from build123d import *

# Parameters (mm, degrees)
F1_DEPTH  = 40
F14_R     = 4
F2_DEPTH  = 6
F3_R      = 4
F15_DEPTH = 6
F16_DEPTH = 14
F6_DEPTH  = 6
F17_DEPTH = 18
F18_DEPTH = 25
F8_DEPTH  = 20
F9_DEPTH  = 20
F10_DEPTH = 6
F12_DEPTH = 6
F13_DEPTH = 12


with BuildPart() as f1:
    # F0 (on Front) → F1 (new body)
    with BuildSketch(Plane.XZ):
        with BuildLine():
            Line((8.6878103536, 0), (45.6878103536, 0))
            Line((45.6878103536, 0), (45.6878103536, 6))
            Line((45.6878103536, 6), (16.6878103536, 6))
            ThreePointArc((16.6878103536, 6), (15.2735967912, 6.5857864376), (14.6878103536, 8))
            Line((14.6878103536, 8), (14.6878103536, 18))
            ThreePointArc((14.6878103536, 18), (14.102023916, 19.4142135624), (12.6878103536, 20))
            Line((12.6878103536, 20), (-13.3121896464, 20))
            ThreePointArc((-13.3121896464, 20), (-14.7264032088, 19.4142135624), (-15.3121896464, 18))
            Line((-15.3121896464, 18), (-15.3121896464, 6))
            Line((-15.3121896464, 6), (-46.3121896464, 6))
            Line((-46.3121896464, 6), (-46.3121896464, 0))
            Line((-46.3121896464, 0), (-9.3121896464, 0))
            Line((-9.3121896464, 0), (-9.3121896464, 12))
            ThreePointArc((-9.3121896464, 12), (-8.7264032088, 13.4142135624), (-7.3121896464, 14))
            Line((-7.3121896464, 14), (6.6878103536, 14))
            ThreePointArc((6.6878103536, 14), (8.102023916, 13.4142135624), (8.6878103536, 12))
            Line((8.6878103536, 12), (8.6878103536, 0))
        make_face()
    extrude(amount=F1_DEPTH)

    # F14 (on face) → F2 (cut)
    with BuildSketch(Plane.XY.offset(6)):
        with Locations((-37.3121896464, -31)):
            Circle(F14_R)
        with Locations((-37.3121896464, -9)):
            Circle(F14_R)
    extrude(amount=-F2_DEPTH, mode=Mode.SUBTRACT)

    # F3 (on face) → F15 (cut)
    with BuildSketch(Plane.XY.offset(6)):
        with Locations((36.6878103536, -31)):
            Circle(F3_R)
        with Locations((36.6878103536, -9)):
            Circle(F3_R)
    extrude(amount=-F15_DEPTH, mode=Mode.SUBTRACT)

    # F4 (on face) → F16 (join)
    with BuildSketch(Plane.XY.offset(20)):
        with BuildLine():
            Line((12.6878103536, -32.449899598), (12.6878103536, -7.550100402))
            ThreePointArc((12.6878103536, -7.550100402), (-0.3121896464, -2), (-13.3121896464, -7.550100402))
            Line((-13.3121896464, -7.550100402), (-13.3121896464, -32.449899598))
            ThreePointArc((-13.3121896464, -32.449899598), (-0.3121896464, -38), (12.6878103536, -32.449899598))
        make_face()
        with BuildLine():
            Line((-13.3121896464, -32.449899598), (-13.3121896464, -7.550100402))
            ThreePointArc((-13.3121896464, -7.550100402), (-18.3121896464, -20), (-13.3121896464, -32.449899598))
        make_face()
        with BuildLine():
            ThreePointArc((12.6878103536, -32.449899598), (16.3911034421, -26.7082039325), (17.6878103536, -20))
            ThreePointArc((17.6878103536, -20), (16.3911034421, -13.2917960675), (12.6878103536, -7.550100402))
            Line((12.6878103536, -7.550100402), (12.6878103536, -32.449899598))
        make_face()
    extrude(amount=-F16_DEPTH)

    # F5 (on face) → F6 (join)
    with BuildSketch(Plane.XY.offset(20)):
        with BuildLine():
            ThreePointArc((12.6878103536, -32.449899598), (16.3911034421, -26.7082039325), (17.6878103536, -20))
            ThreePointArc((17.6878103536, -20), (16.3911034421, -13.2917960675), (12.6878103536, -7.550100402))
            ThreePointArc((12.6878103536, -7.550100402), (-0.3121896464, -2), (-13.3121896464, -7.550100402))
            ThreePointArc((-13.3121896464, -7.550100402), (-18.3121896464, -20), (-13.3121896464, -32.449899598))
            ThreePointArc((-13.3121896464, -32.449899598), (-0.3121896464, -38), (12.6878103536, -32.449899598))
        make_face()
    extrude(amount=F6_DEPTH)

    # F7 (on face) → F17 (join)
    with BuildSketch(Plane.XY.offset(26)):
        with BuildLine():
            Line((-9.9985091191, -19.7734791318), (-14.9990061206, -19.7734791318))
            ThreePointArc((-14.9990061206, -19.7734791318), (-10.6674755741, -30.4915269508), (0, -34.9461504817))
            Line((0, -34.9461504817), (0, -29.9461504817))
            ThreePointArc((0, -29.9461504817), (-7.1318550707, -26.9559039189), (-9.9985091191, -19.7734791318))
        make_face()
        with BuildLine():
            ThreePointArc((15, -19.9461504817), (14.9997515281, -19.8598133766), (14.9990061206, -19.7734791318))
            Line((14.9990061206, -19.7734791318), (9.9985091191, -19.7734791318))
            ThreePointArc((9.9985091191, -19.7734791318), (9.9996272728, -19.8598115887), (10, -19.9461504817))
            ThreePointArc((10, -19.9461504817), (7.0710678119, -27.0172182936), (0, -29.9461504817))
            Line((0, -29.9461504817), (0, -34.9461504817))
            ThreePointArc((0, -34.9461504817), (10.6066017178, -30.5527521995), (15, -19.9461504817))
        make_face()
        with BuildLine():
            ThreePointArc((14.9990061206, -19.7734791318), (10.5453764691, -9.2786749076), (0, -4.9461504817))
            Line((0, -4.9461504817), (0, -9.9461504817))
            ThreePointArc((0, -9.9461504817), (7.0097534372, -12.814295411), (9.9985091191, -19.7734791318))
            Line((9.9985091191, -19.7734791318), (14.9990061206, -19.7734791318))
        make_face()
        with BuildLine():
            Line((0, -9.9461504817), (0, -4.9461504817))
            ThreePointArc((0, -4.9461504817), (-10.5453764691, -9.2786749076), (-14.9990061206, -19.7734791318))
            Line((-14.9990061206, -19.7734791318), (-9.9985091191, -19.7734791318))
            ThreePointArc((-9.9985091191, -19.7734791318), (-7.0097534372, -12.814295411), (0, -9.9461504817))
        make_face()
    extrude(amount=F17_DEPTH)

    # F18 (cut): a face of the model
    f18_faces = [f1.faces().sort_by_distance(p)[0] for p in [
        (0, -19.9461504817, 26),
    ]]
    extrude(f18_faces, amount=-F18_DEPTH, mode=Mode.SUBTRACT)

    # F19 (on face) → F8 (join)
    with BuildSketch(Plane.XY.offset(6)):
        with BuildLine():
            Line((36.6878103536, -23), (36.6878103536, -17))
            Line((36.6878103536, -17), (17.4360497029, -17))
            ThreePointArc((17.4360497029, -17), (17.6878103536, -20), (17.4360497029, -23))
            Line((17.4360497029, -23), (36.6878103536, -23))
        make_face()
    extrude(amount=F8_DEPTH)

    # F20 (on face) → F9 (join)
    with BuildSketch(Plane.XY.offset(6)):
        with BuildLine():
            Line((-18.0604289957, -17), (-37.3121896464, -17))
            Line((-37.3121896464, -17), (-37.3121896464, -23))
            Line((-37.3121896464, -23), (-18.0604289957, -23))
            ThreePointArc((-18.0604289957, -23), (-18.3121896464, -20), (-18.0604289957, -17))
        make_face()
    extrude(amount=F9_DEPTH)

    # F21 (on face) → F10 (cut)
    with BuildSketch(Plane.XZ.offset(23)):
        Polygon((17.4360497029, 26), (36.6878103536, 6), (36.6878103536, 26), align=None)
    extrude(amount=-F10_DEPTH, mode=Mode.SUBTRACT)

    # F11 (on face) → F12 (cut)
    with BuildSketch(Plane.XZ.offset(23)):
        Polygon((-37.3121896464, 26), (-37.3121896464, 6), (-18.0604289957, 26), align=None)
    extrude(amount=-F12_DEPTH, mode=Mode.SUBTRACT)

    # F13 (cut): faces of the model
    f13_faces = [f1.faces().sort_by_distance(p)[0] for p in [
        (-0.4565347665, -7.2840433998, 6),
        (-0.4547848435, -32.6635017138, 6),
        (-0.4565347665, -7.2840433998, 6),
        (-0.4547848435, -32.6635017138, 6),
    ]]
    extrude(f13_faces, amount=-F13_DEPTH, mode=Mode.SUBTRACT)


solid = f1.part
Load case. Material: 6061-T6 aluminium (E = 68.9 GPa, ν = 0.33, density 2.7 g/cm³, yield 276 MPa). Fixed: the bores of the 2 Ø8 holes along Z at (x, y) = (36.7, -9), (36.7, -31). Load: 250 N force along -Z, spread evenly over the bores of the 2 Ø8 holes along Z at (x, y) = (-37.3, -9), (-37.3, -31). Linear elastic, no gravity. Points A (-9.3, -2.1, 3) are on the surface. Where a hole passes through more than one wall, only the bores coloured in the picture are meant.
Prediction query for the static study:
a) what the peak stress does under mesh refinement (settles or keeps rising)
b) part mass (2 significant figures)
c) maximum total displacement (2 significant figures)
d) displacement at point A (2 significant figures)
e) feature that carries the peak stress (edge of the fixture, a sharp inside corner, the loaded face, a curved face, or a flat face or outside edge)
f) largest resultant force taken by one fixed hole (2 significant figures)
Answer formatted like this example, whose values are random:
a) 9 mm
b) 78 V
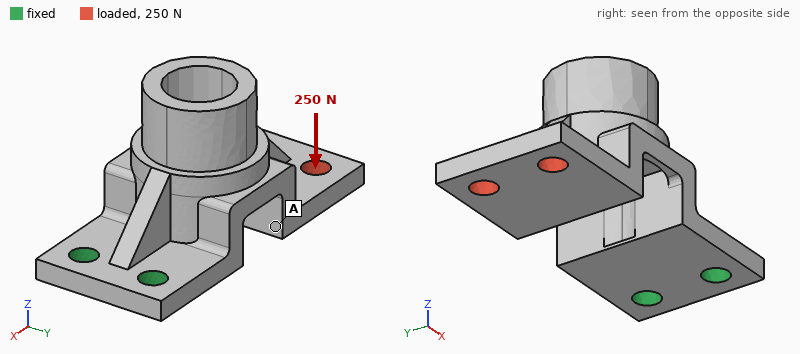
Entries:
a) keeps rising
b) 110 g
c) 0.31 mm
d) 0.13 mm
e) edge of the fixture
f) 150 N
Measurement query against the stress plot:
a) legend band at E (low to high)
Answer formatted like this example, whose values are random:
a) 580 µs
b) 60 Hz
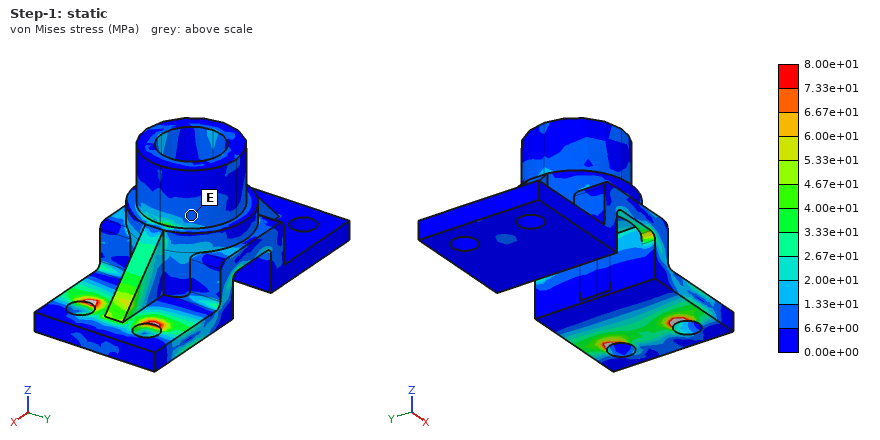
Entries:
a) 6.67e+00 to 1.33e+01 MPa
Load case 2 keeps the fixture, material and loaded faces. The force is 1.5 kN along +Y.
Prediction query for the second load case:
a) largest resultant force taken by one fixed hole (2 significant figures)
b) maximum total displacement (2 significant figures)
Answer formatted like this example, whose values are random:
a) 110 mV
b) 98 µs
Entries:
a) 4.1 kN
b) 0.63 mm
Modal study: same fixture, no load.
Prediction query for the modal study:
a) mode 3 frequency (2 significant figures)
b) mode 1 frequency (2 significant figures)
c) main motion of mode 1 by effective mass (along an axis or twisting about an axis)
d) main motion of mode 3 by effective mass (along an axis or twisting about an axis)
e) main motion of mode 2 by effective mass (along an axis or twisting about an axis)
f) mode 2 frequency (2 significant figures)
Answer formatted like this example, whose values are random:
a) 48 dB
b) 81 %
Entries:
a) 2500 Hz
b) 890 Hz
c) along Z
d) along Y
e) along Y
f) 1700 Hz
